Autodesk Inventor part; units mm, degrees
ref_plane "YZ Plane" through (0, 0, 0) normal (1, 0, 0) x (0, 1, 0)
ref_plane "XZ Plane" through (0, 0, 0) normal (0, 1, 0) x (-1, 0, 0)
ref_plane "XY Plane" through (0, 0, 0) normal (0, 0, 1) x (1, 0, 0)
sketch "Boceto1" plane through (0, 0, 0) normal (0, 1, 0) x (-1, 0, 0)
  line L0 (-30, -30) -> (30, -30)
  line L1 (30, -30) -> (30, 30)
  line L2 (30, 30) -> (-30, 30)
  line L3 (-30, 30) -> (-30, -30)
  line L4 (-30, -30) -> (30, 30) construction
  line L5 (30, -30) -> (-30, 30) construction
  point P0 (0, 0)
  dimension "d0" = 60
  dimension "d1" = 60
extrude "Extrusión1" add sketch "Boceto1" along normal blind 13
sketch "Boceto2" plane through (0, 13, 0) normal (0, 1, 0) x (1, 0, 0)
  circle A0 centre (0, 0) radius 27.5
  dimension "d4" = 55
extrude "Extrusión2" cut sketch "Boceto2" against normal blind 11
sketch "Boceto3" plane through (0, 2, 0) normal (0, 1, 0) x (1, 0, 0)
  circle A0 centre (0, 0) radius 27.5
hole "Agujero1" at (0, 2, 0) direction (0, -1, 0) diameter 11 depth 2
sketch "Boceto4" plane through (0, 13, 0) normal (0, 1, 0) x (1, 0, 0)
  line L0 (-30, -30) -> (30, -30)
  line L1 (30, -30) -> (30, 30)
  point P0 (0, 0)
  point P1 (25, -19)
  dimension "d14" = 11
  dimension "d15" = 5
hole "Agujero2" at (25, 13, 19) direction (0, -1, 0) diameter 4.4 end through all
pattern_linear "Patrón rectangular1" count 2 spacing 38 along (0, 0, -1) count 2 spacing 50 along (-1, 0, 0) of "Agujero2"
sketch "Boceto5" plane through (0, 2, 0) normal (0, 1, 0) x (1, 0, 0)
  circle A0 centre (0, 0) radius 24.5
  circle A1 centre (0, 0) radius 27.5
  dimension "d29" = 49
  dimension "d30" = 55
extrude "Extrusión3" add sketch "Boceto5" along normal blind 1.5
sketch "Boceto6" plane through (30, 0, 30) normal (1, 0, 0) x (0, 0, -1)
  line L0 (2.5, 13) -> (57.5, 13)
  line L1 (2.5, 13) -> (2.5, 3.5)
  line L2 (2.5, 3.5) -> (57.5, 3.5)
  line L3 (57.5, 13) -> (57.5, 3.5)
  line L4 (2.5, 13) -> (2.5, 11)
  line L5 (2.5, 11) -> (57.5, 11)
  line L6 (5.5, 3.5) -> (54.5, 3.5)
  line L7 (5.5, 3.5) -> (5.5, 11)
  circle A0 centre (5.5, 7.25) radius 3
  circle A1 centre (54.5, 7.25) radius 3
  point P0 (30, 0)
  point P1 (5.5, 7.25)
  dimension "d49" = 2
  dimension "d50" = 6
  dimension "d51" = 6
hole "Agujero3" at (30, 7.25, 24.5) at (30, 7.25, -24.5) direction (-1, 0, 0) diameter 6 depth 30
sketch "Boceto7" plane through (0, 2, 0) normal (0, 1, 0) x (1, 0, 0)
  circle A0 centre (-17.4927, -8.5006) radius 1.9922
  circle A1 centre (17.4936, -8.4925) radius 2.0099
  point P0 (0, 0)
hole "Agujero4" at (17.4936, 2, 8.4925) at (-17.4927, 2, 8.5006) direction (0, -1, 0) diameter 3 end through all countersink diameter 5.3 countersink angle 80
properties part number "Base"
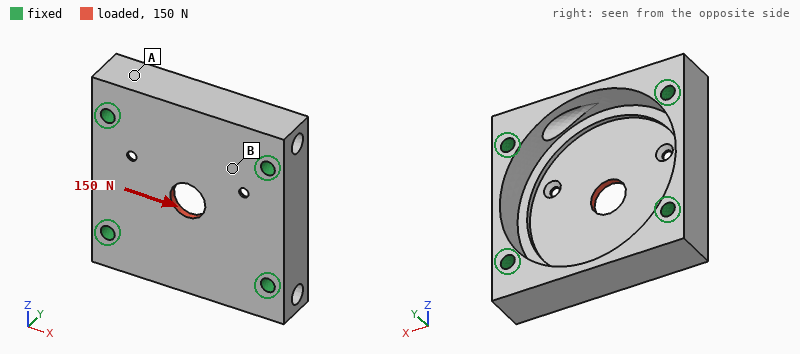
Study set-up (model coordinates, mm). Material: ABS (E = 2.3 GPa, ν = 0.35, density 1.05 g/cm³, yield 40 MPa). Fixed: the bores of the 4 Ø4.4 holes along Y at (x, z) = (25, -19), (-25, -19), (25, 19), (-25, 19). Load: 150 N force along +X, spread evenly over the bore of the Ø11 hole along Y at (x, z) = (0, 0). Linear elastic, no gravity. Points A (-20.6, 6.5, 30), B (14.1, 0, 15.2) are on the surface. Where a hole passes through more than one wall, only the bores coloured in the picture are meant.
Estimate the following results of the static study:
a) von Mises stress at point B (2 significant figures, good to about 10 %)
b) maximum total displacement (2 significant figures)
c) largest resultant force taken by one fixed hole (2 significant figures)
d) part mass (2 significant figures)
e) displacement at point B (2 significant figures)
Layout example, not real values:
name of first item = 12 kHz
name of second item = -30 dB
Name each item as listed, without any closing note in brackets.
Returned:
von Mises stress at point B = 0.89 MPa
maximum total displacement = 19 µm
largest resultant force taken by one fixed hole = 42 N
part mass = 20 g
displacement at point B = 6.5 µm
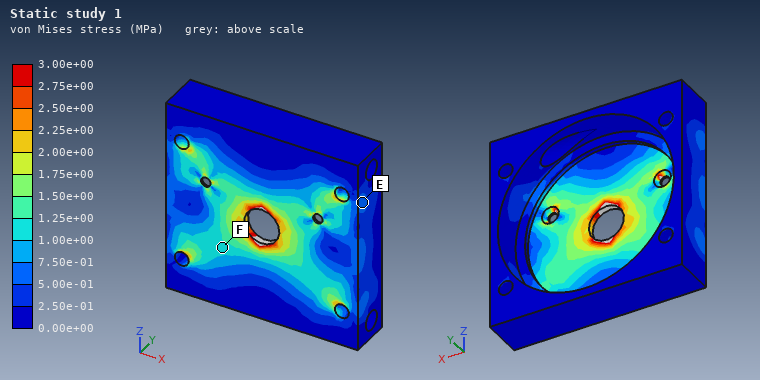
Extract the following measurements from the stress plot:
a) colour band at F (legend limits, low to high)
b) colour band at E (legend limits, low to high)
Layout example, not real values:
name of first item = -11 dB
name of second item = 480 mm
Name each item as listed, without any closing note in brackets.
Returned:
colour band at F = 1.00e+00 to 1.25e+00 MPa
colour band at E = 5.00e-01 to 7.50e-01 MPa
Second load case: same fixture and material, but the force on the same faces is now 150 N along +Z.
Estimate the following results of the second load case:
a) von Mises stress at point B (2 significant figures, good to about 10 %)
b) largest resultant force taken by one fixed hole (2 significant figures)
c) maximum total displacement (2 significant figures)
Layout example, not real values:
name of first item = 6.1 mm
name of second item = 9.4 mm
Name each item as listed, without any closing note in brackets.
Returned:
von Mises stress at point B = 1.1 MPa
largest resultant force taken by one fixed hole = 40 N
maximum total displacement = 23 µm
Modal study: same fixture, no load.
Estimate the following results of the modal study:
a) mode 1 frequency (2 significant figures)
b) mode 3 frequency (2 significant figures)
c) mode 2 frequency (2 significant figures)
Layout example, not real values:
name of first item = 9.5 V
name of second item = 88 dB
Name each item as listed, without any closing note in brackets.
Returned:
mode 1 frequency = 2100 Hz
mode 3 frequency = 3900 Hz
mode 2 frequency = 3700 Hz
